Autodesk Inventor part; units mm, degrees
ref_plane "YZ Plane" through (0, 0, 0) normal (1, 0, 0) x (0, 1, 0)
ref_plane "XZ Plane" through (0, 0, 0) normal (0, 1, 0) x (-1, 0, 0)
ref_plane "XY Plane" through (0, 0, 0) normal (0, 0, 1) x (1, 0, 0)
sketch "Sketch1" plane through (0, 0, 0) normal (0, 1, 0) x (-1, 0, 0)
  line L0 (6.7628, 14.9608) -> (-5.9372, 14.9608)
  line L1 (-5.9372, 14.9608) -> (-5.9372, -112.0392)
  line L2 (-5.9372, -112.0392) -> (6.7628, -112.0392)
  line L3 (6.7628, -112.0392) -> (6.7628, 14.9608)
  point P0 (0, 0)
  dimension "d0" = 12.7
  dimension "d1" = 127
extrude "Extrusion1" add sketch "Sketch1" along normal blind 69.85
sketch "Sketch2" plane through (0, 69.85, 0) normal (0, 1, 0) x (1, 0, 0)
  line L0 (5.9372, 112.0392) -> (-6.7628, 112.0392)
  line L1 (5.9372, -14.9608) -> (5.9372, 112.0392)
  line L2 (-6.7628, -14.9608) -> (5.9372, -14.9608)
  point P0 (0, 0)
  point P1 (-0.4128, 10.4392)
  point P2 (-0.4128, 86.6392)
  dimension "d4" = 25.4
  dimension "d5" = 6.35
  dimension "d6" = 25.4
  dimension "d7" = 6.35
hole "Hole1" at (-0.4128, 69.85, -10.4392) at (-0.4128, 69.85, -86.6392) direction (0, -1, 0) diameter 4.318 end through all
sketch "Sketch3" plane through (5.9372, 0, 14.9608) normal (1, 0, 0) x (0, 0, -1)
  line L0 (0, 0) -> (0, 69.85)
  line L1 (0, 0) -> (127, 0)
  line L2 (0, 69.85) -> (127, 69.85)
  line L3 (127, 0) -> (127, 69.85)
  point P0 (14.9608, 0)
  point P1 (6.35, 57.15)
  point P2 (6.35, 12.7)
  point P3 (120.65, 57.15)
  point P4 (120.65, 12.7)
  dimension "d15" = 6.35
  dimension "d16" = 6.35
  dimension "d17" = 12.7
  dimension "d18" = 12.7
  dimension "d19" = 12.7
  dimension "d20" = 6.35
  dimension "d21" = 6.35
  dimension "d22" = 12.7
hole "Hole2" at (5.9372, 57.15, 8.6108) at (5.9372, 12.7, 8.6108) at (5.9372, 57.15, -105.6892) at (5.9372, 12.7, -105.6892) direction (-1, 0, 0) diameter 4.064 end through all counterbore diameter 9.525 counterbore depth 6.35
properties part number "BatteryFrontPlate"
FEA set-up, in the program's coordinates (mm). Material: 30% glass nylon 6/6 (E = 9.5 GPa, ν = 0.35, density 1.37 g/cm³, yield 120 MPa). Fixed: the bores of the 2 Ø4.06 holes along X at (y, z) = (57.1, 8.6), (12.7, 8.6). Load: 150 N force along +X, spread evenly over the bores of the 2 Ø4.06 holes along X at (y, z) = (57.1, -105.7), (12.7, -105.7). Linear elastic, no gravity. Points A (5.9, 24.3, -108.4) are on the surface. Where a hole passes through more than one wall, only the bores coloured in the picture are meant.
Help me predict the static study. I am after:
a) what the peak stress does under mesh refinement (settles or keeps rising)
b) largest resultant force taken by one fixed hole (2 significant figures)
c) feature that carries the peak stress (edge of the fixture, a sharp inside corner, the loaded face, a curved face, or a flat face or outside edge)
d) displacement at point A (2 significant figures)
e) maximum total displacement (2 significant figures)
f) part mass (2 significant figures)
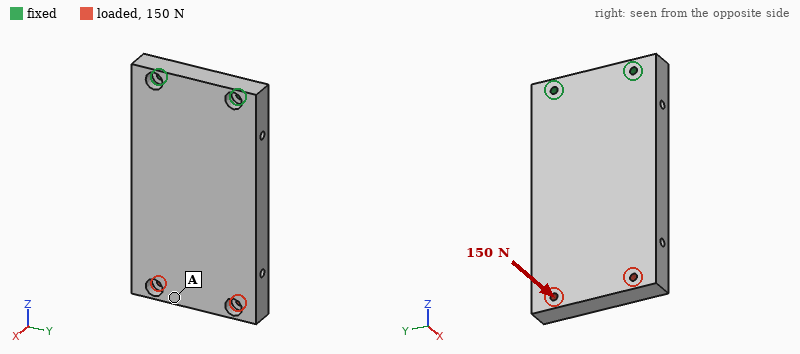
keeps rising
90 N
edge of the fixture
1.5 mm
1.6 mm
150 g
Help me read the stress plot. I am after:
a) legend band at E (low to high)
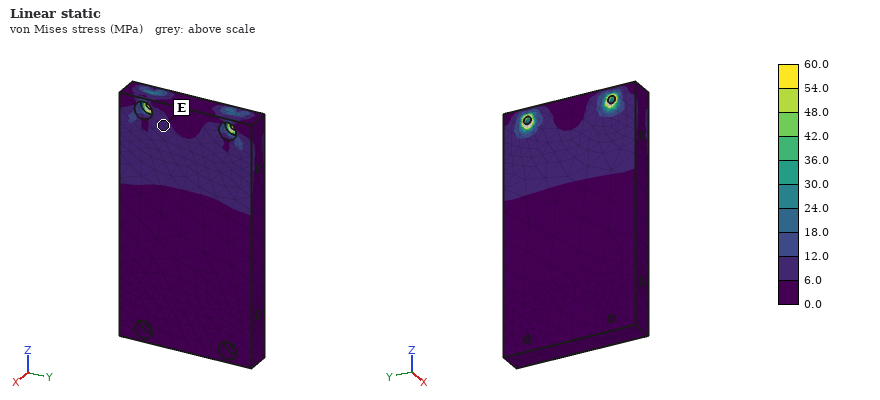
6.0 to 12.0 MPa
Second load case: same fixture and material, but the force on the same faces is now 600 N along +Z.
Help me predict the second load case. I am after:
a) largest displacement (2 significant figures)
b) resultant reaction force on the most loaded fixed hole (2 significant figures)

0.12 mm
300 N
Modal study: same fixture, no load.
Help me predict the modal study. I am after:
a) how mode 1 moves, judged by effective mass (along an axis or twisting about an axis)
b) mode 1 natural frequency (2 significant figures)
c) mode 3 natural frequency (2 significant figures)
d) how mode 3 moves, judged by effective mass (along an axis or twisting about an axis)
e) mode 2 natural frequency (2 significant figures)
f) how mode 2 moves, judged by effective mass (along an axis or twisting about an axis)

along X
240 Hz
1300 Hz
along Y
1100 Hz
along Y
